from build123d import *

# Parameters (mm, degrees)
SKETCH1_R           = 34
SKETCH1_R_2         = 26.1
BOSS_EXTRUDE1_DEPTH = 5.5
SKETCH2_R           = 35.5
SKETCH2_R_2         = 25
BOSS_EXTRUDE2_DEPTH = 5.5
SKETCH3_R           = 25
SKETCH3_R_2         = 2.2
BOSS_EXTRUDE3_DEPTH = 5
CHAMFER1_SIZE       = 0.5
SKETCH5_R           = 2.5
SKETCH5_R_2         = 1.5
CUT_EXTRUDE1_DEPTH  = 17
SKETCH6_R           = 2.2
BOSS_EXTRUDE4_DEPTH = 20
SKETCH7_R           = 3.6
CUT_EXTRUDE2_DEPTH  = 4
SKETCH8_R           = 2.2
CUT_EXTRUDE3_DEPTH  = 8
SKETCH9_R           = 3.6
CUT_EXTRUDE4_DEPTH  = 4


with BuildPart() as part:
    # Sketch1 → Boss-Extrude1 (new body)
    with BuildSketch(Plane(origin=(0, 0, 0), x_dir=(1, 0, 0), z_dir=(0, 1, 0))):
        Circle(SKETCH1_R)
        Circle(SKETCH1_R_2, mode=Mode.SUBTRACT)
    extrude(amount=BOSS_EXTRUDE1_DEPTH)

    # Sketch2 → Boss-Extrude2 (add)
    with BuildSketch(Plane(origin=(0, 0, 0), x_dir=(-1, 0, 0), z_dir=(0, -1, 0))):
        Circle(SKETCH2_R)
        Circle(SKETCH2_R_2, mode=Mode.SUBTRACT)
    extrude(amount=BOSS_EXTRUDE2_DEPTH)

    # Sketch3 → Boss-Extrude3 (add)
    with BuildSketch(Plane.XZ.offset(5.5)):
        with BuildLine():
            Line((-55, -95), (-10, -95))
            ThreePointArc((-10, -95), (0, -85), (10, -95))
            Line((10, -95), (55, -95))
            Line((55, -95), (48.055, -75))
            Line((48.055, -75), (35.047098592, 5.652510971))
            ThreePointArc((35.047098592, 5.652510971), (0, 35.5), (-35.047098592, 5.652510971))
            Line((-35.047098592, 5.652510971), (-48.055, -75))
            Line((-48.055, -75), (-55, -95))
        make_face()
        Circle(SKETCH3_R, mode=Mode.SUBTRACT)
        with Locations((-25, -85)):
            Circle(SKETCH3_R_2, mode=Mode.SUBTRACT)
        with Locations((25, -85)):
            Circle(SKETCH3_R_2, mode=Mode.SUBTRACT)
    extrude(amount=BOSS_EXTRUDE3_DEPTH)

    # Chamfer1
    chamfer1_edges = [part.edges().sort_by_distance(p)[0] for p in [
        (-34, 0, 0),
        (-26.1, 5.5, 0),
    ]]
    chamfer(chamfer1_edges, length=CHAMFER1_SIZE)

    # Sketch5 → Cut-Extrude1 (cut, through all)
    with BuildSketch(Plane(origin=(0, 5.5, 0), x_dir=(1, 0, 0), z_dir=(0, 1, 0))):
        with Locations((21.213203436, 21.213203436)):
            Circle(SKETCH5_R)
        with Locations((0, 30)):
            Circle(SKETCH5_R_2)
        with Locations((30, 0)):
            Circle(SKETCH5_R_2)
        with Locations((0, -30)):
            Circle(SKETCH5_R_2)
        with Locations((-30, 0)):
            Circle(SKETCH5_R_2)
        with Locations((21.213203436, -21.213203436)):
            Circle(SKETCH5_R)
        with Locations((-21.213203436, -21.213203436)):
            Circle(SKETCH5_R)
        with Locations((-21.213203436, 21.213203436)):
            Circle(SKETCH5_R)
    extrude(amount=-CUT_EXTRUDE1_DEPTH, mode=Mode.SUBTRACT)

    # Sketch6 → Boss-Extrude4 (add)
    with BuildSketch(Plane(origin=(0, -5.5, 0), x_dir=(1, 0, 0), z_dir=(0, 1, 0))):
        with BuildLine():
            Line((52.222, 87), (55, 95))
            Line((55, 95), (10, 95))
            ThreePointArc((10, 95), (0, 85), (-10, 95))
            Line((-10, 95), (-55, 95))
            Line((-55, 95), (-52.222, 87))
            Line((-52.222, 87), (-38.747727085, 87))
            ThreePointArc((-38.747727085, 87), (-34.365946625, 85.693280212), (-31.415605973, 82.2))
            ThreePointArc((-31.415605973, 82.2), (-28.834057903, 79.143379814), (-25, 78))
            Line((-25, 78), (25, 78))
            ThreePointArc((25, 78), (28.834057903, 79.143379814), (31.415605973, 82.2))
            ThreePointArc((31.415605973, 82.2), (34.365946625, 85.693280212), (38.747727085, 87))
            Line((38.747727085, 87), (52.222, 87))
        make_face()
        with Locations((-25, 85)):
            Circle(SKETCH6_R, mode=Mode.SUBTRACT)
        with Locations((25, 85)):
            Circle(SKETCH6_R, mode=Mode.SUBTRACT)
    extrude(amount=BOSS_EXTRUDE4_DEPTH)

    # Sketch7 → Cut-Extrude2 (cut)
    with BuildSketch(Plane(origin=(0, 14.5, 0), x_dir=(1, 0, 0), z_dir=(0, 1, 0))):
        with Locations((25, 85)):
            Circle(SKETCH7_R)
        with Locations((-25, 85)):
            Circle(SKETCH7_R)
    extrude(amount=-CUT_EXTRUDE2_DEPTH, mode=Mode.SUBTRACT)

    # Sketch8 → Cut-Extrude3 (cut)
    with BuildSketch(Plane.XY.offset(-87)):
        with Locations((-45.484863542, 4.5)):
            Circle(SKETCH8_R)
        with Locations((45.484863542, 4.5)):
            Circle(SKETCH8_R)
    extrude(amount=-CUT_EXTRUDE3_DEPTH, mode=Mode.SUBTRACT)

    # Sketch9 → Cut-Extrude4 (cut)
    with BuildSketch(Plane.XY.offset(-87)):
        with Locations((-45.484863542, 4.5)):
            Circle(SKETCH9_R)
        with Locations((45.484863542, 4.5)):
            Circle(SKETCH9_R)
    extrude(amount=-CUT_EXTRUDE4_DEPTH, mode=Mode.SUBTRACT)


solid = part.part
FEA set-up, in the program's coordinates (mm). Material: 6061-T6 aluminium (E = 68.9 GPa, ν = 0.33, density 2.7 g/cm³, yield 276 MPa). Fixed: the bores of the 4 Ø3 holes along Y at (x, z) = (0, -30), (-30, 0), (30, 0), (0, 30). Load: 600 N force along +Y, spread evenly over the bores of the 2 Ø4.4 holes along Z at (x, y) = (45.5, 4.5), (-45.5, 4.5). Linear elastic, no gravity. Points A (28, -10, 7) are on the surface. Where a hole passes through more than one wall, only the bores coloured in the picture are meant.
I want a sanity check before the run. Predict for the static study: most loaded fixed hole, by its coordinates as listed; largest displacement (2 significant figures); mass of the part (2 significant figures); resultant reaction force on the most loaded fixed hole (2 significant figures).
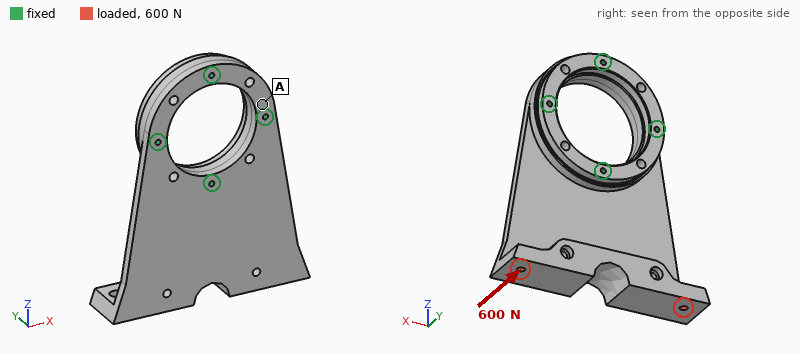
(0, -30)
0.93 mm
220 g
1.2 kN
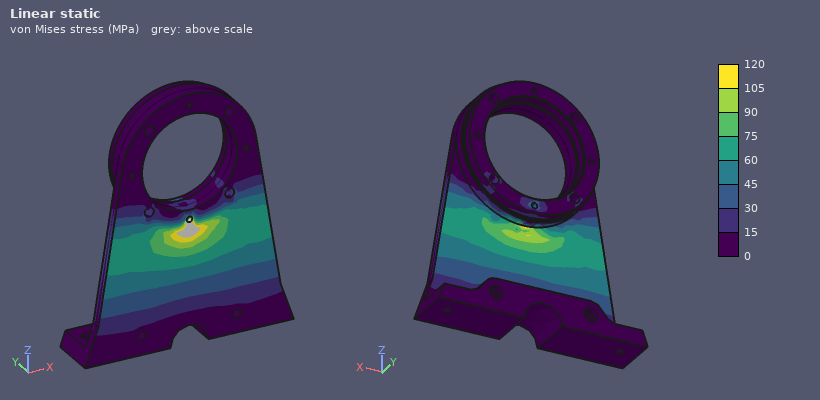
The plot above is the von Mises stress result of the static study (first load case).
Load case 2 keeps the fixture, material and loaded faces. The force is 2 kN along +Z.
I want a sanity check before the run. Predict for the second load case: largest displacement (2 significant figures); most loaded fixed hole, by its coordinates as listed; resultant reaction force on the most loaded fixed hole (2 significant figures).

0.90 mm
(0, -30)
1.1 kN
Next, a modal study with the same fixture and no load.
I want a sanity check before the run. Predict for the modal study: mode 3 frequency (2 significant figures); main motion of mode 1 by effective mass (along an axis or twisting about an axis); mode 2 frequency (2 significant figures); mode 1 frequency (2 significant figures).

2800 Hz
along Y
900 Hz
490 Hz
